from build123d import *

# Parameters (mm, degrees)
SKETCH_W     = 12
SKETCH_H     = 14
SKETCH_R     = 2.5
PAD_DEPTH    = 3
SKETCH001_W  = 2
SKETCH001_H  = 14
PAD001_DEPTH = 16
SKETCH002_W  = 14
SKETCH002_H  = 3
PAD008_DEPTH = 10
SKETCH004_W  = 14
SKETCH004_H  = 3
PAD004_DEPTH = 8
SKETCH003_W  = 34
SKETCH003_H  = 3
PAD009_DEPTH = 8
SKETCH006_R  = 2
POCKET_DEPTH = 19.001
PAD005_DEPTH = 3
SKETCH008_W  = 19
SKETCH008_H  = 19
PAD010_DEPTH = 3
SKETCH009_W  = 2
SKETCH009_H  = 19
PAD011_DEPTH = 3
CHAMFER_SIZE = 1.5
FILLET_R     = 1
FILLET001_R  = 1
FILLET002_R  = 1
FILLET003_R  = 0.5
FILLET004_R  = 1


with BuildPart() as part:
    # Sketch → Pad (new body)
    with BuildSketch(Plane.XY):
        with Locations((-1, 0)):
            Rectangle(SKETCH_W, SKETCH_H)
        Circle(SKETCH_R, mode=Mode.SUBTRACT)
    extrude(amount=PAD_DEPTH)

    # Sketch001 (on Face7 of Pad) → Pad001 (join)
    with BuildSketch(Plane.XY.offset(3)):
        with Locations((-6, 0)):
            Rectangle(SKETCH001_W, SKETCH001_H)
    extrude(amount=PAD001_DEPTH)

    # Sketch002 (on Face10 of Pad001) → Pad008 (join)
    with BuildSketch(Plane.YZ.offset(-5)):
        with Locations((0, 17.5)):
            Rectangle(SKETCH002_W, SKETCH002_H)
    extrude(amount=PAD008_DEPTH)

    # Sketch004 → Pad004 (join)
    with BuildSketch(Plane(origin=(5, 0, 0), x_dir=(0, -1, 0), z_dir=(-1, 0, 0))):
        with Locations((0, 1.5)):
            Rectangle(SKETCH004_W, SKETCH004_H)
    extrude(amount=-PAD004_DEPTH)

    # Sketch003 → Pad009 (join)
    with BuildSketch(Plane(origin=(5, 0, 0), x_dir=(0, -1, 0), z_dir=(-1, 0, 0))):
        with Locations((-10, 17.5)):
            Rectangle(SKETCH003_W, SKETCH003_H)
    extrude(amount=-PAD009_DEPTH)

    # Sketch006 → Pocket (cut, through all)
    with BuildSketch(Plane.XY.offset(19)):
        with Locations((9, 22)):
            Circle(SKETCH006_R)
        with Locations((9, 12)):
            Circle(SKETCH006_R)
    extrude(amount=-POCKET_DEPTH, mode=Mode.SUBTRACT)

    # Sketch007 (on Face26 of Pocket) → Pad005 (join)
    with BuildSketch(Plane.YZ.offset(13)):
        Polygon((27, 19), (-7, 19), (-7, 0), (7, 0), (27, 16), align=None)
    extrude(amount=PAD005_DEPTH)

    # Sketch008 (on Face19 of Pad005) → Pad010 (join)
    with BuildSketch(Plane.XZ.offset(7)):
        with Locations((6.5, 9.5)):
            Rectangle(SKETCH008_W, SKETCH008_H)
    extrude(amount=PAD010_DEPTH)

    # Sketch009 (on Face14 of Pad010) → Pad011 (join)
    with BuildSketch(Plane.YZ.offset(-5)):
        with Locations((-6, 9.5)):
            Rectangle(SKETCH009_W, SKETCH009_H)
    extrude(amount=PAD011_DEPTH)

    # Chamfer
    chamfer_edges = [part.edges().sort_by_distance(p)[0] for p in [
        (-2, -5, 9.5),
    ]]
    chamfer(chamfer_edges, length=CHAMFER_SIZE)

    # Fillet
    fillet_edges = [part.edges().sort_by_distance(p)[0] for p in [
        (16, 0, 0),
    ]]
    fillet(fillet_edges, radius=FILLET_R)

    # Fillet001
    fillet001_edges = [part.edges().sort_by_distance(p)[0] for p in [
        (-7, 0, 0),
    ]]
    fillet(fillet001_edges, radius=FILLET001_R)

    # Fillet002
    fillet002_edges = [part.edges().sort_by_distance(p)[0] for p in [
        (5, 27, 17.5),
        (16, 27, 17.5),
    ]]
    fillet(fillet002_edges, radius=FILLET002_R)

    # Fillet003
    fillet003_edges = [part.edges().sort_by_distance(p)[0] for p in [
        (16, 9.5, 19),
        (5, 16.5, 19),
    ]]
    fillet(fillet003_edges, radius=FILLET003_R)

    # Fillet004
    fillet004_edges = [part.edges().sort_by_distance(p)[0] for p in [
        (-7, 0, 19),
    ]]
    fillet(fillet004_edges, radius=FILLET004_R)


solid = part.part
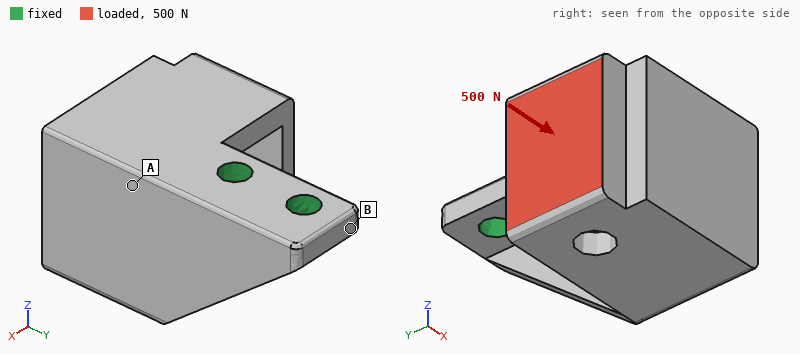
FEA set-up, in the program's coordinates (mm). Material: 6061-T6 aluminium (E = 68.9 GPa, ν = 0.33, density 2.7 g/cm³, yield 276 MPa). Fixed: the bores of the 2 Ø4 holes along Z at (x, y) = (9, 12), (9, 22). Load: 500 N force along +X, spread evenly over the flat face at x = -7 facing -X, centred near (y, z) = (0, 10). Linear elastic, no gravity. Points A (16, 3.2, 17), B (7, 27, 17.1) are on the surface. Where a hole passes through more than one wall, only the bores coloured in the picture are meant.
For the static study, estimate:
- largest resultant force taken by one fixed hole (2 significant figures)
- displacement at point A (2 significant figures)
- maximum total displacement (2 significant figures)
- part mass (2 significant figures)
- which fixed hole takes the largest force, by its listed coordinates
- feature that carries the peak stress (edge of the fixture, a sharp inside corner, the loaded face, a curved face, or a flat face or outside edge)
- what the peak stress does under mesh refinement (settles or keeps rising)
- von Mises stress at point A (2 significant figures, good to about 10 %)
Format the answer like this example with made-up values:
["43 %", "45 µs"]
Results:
["780 N", "0.042 mm", "0.21 mm", "13 g", "(9, 12)", "edge of the fixture", "keeps rising", "36 MPa"]
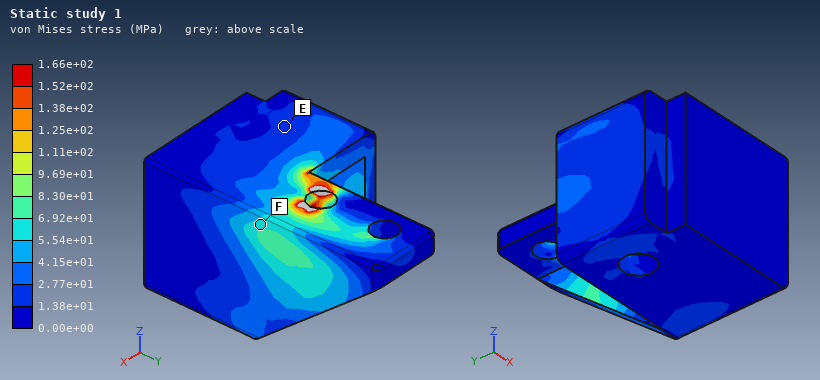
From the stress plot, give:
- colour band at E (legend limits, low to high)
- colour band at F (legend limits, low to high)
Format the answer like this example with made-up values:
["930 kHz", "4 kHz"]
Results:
["1.38e+01 to 2.77e+01 MPa", "5.54e+01 to 6.92e+01 MPa"]
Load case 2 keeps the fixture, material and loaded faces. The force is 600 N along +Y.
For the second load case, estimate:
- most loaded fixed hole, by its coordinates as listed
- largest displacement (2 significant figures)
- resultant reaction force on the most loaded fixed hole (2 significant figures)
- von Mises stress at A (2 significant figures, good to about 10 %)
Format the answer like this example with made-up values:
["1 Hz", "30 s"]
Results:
["(9, 12)", "0.23 mm", "1.0 kN", "80 MPa"]
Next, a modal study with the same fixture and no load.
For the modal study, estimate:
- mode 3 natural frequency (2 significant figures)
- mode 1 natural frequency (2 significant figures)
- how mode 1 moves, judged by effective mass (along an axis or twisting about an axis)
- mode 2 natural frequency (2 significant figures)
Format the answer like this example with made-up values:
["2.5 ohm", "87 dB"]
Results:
["6700 Hz", "2500 Hz", "along X", "3600 Hz"]
